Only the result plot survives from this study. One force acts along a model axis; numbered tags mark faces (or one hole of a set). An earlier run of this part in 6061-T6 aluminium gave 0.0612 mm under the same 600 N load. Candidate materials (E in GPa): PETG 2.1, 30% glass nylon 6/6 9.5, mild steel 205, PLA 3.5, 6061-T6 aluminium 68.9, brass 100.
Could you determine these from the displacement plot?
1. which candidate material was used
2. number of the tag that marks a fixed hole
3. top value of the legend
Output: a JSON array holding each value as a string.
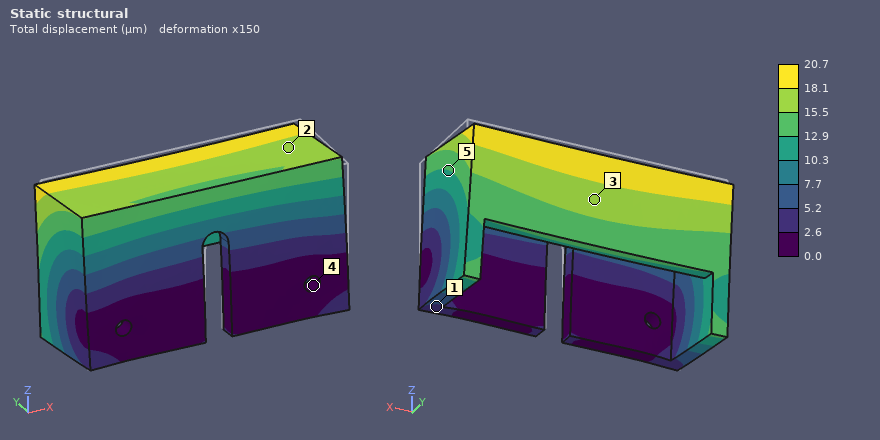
["mild steel", "4", "20.7 µm"]
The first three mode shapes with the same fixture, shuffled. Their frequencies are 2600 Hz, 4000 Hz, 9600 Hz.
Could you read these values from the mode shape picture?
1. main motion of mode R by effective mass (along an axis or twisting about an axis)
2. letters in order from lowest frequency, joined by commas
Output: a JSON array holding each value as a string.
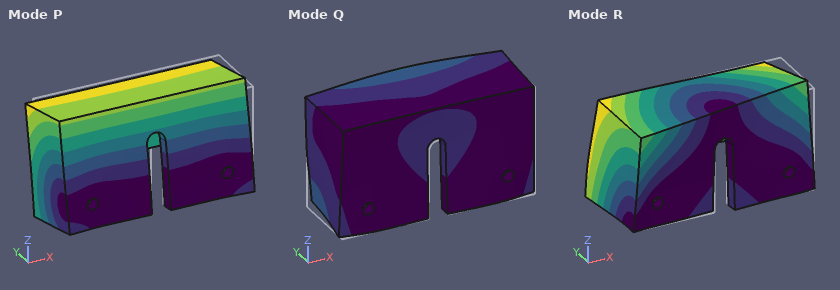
["along X", "P, R, Q"]
